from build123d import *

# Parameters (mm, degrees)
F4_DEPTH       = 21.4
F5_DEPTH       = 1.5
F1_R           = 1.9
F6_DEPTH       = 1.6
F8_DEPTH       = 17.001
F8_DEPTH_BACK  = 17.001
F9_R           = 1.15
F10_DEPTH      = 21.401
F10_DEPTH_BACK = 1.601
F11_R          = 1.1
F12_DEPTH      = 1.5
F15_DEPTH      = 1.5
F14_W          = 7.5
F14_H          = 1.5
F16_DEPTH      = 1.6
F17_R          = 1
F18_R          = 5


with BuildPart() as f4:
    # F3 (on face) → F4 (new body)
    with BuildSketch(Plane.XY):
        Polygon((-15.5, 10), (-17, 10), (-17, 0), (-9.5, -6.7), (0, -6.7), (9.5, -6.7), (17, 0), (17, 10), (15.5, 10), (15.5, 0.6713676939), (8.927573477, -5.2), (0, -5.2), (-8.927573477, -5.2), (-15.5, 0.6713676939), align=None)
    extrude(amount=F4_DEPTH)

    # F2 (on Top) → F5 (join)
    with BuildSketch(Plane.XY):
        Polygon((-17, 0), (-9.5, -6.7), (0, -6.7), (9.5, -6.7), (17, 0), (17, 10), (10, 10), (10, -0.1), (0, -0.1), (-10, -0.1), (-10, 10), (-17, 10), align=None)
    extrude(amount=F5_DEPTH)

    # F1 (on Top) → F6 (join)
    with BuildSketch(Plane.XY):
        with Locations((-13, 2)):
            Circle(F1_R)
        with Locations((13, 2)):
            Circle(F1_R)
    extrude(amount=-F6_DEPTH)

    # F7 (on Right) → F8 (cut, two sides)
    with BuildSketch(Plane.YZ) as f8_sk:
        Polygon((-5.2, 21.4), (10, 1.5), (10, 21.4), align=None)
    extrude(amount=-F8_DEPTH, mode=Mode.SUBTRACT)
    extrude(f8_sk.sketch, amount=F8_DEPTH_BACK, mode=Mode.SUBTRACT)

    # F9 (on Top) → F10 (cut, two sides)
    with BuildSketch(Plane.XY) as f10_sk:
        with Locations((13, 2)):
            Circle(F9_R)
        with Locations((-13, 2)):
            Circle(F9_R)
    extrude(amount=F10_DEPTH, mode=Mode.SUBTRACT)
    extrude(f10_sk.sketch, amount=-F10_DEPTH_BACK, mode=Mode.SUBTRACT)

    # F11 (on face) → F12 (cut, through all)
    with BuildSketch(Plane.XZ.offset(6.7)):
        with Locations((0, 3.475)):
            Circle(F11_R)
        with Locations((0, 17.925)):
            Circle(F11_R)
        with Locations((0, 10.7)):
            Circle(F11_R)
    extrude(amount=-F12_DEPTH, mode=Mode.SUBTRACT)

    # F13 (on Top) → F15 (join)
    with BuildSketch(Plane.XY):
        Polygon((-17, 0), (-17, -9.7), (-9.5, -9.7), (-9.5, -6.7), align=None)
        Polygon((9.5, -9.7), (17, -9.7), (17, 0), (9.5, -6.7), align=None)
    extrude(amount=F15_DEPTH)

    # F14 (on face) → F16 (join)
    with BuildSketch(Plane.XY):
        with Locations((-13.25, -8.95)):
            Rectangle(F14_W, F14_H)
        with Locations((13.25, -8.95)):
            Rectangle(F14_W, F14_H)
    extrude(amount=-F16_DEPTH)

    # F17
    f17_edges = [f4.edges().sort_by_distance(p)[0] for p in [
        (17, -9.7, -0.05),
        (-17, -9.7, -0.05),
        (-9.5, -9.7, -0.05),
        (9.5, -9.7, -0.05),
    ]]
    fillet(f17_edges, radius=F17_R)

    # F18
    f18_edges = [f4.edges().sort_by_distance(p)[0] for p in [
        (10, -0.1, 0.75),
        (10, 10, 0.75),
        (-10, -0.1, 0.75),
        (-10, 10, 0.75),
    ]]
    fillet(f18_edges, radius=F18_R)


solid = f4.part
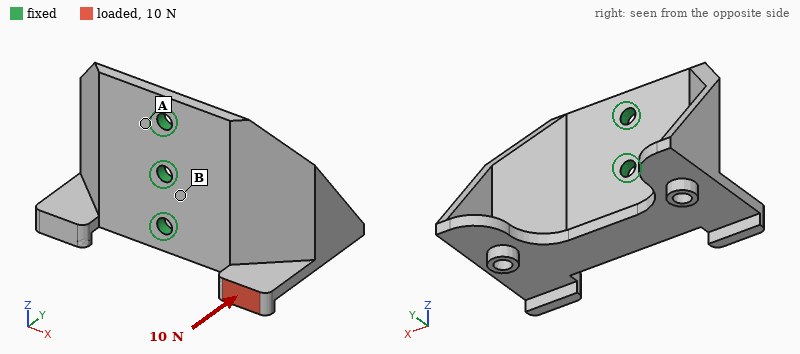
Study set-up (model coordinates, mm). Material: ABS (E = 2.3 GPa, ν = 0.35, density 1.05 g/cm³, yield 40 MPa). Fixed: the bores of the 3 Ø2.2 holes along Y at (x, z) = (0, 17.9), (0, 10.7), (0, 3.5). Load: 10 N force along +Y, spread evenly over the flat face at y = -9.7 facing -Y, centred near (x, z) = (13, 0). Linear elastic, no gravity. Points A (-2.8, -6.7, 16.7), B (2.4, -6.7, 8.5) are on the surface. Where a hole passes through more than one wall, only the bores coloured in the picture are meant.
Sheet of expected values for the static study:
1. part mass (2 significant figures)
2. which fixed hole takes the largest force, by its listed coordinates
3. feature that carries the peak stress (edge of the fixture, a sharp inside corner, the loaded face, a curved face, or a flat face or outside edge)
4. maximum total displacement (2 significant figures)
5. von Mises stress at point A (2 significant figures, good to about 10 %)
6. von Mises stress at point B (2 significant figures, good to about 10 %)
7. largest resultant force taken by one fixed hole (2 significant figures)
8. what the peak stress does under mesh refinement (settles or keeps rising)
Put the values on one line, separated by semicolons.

1.9 g; (0, 3.5); edge of the fixture; 0.52 mm; 2.0 MPa; 5.5 MPa; 11 N; keeps rising
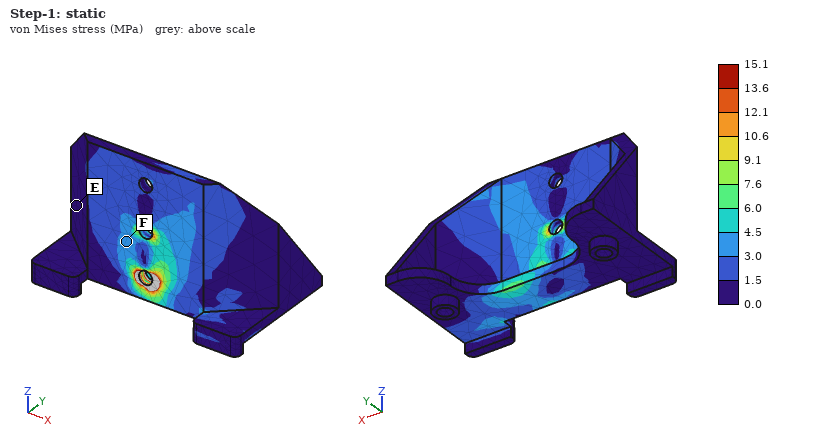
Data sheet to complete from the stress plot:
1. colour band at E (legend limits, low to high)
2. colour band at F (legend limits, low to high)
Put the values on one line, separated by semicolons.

0.0 to 1.5 MPa; 3.0 to 4.5 MPa
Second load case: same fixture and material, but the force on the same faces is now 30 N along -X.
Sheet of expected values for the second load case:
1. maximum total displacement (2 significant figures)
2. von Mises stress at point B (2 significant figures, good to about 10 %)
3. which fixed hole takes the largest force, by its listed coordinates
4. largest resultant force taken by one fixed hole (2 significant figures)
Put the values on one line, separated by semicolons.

0.52 mm; 5.8 MPa; (0, 3.5); 33 N
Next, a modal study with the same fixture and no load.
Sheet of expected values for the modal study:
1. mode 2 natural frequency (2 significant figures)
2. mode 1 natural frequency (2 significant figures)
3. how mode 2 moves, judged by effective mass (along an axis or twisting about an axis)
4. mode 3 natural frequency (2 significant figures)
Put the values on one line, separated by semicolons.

1700 Hz; 900 Hz; along Y; 1800 Hz
